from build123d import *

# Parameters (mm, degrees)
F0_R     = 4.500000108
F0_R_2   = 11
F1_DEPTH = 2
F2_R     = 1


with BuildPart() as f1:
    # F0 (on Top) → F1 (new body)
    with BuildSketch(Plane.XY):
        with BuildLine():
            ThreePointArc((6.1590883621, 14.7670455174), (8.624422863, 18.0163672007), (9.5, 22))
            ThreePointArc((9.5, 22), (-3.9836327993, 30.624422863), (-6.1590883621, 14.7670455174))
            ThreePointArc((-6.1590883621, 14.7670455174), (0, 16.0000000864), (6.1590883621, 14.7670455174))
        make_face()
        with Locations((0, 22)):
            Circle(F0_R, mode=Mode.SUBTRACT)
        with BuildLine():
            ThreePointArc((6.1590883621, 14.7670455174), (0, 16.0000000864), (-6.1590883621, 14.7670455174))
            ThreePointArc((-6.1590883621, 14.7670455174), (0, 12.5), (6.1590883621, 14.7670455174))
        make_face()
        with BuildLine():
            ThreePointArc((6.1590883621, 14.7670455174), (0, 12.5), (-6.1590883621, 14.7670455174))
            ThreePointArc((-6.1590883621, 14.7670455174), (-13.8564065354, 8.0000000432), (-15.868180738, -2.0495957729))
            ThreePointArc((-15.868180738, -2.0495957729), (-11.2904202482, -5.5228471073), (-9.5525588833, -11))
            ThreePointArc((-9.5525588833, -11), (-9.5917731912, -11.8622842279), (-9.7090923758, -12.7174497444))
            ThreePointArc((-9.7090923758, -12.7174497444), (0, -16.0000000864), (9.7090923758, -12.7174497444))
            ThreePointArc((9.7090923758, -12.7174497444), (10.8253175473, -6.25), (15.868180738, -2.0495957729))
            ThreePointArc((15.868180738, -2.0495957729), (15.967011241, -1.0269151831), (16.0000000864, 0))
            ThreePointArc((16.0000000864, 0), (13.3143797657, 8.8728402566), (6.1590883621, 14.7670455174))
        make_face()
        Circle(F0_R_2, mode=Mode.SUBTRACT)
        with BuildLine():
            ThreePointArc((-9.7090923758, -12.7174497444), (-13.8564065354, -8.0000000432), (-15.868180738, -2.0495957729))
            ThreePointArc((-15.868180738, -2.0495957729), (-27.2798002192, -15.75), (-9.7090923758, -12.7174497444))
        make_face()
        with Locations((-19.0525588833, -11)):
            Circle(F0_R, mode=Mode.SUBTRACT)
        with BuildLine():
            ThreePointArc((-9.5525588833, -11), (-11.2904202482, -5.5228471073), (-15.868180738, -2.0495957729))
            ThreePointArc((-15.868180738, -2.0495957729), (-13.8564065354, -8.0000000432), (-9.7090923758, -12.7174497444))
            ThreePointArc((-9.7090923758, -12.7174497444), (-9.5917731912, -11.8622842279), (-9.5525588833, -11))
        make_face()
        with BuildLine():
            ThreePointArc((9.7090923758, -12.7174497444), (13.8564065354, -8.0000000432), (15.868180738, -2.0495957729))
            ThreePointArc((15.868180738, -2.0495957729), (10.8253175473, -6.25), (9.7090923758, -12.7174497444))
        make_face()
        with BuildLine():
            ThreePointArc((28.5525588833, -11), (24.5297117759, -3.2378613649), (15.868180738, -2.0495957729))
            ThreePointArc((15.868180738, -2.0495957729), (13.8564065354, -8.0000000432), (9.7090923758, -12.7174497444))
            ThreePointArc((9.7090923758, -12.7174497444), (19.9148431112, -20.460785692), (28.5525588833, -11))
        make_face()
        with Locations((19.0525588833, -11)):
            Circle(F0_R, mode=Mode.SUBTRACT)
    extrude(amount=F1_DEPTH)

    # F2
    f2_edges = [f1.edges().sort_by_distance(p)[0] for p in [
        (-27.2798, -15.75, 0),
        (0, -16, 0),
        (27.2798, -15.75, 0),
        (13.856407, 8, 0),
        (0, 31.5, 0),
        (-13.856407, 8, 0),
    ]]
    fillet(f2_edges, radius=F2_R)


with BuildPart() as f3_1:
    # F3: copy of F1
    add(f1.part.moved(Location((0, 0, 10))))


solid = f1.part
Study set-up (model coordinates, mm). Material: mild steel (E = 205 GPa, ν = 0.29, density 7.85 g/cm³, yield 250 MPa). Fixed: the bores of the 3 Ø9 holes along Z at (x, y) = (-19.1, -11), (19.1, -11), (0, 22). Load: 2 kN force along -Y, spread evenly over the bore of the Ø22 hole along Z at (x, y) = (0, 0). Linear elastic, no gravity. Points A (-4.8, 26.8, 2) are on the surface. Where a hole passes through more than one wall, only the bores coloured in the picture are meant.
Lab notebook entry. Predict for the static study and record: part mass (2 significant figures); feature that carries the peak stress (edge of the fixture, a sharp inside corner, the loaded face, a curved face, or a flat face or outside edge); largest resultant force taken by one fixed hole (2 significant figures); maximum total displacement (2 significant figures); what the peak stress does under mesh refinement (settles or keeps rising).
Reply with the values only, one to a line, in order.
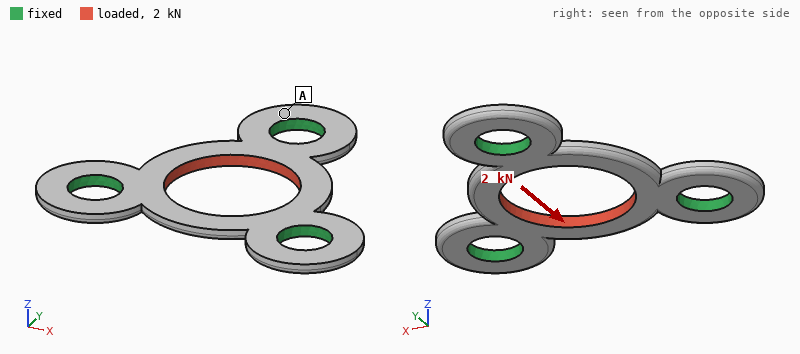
15 g
a sharp inside corner
730 N
7.0 µm
keeps rising
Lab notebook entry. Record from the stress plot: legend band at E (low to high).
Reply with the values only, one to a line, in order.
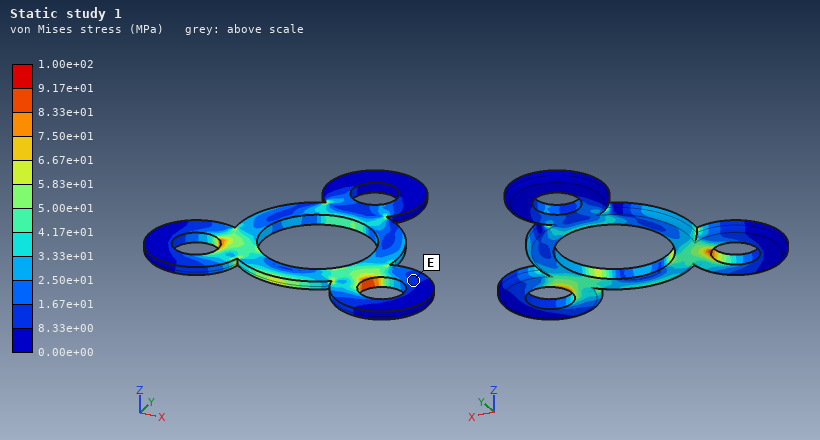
8.33e+00 to 1.67e+01 MPa
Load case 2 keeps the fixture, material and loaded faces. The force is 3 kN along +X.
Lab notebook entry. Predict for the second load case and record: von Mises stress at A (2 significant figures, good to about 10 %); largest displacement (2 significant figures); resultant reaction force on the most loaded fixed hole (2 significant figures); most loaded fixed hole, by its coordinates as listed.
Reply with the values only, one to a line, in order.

11 MPa
9.2 µm
1.2 kN
(0, 22)
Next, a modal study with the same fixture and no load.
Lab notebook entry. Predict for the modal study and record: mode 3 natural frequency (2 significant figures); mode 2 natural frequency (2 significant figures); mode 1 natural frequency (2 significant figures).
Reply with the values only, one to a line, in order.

13 kHz
13 kHz
13 kHz
